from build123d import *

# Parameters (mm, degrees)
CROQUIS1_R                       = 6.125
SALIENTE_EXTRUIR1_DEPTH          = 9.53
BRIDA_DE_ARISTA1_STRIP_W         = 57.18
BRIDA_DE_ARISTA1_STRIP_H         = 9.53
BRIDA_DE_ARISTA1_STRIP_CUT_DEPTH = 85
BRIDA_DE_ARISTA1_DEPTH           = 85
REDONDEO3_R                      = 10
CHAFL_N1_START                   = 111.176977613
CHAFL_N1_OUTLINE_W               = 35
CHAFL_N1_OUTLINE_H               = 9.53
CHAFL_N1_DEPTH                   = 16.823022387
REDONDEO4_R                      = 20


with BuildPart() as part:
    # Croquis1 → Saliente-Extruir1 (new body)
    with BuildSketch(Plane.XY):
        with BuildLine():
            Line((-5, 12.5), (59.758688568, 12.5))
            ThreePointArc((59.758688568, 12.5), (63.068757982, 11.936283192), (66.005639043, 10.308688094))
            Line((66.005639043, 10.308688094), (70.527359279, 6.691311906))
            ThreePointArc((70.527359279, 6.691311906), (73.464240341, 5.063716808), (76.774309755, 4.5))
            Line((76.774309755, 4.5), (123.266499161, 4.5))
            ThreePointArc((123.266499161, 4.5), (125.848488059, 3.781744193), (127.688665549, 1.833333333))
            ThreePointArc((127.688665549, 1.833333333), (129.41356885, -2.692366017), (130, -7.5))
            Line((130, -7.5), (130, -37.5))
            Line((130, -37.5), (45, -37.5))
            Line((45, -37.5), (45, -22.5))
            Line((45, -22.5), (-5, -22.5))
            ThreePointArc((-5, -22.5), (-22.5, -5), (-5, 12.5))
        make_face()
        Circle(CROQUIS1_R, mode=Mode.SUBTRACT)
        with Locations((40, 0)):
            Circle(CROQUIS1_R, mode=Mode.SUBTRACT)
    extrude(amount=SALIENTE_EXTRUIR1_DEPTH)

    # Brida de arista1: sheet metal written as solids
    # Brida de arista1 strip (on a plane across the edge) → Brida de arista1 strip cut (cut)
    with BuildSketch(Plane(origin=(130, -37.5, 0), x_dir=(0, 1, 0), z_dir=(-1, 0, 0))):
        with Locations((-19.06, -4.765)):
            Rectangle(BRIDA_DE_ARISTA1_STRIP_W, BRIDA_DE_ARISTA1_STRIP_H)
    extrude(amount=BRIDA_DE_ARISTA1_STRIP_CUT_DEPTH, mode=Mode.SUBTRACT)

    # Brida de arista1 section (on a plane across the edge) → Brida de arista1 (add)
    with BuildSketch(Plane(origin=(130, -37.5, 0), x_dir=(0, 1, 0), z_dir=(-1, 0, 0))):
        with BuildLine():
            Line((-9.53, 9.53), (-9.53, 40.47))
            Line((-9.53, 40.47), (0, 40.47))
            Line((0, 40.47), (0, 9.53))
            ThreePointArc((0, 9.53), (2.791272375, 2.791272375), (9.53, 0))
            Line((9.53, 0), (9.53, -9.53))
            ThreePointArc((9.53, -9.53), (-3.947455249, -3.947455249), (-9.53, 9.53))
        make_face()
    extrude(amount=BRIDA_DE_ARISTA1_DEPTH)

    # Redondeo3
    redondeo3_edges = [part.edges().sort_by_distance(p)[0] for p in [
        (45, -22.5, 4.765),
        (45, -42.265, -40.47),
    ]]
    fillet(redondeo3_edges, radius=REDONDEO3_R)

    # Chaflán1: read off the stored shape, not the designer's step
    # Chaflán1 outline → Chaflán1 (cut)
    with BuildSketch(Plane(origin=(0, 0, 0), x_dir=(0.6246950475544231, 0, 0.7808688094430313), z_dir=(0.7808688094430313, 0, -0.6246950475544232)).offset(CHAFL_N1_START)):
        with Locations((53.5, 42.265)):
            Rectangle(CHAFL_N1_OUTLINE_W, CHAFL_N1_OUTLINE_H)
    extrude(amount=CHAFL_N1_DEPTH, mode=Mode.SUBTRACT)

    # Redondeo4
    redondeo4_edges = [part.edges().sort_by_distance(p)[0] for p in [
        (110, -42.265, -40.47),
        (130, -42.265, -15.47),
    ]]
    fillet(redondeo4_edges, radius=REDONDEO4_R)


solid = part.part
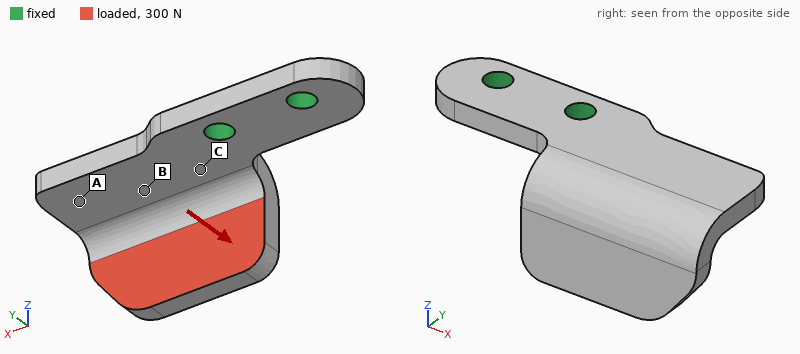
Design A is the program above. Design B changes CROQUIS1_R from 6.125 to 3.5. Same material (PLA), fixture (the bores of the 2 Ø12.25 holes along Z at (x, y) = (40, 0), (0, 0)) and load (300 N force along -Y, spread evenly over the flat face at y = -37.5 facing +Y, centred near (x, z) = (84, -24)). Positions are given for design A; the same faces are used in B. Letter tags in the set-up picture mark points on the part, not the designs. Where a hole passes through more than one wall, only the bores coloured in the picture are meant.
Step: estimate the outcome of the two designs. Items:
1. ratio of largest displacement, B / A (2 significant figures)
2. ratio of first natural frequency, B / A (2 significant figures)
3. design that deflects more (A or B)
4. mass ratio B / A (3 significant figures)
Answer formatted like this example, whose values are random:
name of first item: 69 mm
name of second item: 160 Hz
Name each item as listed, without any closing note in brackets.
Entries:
ratio of largest displacement, B / A: 1.1
ratio of first natural frequency, B / A: 0.91
design that deflects more: B
mass ratio B / A: 1.02
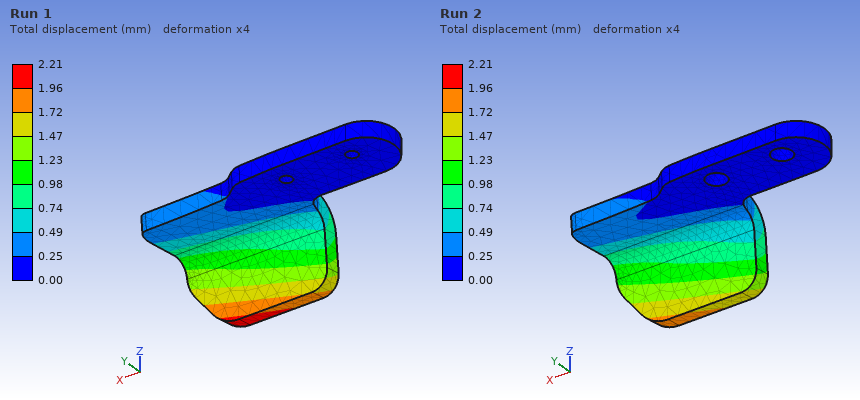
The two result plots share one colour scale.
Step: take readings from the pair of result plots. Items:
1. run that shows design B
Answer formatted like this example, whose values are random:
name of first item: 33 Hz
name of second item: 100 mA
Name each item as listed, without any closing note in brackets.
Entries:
run that shows design B: Run 1
